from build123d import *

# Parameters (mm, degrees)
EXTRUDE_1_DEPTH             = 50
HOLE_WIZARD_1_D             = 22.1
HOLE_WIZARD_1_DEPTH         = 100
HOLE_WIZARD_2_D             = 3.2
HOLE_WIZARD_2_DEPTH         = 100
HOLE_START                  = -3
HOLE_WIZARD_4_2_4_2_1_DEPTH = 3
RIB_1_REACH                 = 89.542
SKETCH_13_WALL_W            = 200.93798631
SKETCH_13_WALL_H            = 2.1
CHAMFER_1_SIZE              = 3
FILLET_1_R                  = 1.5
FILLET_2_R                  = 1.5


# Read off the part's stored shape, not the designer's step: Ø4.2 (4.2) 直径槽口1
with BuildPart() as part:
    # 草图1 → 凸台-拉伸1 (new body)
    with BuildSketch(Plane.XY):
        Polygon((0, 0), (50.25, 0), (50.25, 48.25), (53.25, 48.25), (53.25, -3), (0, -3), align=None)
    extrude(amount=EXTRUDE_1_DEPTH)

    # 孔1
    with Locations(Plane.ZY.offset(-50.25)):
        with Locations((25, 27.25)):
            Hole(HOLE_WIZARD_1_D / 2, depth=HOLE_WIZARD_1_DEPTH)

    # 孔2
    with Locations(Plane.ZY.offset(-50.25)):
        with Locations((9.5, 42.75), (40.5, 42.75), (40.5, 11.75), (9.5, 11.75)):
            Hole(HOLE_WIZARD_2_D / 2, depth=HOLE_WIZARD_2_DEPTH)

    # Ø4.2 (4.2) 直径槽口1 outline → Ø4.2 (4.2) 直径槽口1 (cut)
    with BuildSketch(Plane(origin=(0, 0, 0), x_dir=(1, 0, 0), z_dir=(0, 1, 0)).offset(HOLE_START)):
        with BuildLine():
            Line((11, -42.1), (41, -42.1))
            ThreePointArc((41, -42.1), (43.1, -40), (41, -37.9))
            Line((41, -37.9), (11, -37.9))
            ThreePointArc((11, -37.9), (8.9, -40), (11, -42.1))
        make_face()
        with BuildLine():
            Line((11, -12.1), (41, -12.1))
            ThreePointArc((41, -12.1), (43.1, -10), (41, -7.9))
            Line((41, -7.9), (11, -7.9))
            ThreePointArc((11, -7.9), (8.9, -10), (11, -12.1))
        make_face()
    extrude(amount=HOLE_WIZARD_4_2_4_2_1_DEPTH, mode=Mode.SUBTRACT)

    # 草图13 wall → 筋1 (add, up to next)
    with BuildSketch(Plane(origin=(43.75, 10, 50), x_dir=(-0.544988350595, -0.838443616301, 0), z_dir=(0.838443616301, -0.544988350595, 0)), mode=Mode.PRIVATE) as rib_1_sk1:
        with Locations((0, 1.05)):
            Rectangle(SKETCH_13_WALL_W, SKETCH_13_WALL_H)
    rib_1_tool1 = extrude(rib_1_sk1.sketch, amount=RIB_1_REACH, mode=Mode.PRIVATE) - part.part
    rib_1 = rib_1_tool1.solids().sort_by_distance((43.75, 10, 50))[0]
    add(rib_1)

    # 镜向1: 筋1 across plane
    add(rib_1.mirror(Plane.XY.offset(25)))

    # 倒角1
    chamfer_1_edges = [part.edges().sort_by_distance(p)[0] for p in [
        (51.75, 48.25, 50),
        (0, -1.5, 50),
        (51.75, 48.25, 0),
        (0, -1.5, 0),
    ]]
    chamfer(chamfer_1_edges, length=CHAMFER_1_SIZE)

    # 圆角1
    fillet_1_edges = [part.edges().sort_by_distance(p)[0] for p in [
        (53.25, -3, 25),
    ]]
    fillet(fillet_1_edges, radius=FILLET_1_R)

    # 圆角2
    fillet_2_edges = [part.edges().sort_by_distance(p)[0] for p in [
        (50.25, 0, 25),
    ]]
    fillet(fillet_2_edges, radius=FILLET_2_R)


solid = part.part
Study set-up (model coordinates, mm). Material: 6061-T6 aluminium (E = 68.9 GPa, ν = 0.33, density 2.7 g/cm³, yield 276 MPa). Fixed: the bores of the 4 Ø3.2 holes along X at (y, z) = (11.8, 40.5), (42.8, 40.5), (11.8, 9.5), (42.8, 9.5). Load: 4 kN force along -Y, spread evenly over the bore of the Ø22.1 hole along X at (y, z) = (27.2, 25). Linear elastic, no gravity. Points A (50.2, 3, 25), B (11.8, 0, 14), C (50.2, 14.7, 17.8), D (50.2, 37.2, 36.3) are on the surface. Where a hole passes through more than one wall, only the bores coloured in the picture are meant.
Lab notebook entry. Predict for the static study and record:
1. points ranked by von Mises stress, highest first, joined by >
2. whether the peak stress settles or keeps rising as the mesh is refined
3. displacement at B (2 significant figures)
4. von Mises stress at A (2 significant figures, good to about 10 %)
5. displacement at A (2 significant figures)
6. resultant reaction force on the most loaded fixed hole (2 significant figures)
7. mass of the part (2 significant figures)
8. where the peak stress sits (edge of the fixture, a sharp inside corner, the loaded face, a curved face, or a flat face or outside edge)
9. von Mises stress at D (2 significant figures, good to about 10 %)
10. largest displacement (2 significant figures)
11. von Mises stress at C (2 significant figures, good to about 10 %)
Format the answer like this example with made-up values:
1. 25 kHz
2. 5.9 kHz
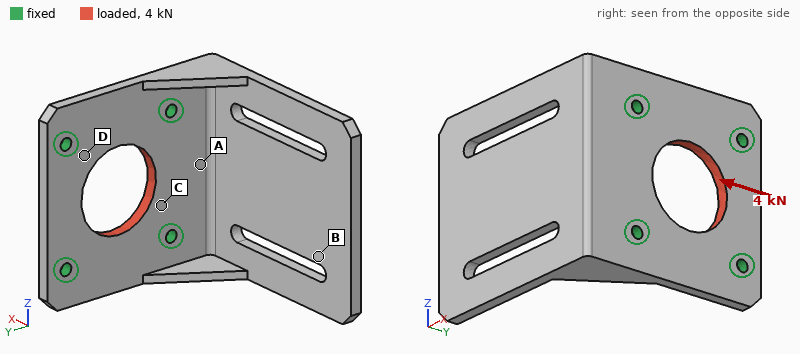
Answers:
1. D > C > A > B
2. keeps rising
3. 5.3 µm
4. 8.1 MPa
5. 4.9 µm
6. 1.0 kN
7. 37 g
8. edge of the fixture
9. 28 MPa
10. 13 µm
11. 17 MPa
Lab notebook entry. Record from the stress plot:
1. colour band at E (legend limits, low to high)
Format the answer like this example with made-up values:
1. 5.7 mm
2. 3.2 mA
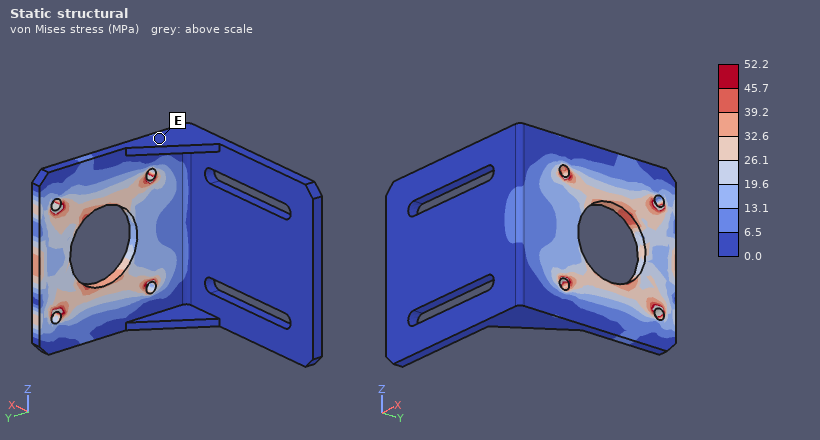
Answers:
1. 0.0 to 6.5 MPa
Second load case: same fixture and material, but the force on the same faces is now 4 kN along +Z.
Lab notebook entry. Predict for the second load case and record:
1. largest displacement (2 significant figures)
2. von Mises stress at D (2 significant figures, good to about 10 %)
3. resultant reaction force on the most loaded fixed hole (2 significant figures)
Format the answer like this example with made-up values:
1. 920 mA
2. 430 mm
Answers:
1. 9.5 µm
2. 23 MPa
3. 1.0 kN
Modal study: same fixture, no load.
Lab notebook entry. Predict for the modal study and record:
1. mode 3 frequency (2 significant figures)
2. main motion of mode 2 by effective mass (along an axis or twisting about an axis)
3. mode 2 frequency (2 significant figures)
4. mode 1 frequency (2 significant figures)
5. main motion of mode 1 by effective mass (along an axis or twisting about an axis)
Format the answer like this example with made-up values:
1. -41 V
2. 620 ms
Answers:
1. 3100 Hz
2. along Z
3. 2000 Hz
4. 890 Hz
5. along Y
